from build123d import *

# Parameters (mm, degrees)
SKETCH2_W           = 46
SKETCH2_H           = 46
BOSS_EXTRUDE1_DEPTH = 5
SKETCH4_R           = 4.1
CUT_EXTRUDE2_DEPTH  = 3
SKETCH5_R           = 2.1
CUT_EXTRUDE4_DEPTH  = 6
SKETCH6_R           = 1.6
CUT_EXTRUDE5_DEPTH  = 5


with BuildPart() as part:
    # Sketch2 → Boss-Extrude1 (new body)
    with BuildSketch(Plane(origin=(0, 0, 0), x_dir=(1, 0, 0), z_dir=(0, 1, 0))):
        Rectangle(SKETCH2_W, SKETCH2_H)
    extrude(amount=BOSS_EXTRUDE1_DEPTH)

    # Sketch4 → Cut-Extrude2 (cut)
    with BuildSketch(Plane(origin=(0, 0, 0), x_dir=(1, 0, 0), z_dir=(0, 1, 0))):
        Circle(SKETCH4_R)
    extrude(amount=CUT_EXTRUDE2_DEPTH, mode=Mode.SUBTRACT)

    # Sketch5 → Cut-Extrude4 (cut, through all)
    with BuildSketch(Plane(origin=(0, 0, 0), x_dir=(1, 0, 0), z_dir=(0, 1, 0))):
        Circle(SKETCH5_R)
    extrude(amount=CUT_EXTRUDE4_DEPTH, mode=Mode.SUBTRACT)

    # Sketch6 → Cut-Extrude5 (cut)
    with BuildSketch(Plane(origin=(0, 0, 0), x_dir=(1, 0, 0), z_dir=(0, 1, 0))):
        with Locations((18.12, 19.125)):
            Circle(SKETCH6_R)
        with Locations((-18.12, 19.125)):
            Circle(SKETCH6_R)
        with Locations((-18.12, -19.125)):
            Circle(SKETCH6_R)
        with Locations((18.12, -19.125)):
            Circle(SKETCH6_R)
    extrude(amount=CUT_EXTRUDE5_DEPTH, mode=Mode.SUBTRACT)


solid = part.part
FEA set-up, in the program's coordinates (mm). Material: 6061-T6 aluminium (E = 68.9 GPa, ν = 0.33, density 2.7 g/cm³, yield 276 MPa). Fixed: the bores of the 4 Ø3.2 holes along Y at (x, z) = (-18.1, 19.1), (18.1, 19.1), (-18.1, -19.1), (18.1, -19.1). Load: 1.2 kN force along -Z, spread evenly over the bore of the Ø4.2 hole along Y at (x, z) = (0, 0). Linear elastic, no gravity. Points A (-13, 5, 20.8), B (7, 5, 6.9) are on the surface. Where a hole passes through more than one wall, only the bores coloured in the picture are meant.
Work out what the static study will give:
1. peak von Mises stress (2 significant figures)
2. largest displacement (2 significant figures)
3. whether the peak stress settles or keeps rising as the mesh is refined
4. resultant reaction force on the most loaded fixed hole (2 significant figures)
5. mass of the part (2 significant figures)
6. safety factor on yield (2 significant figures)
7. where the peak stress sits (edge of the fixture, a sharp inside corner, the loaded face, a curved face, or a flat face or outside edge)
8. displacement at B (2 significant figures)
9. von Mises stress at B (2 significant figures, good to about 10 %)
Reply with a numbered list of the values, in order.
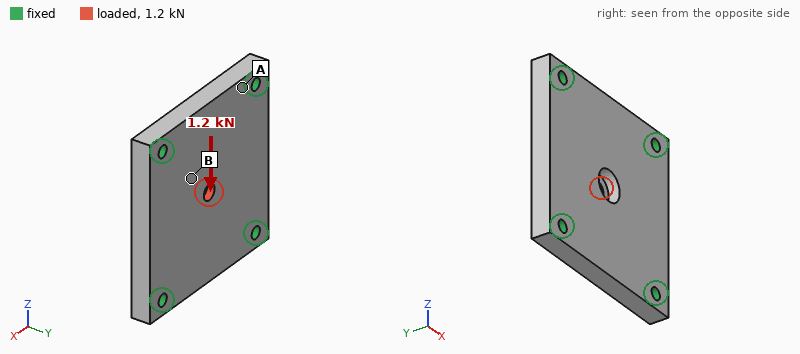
1. 82 MPa
2. 5.3 µm
3. settles
4. 340 N
5. 28 g
6. 3.4
7. the loaded face
8. 2.0 µm
9. 10 MPa
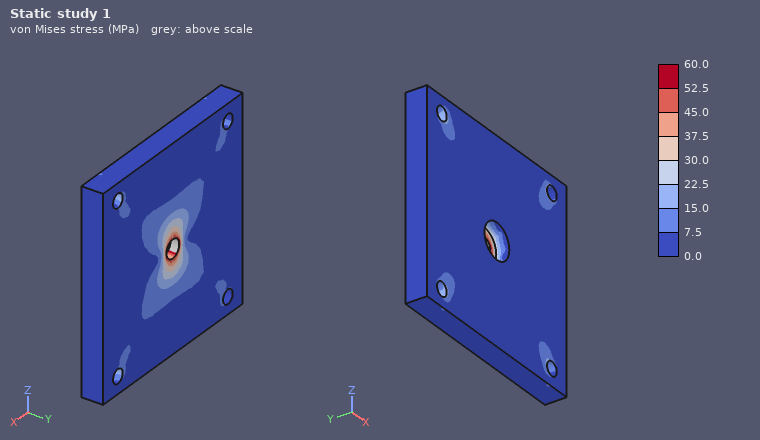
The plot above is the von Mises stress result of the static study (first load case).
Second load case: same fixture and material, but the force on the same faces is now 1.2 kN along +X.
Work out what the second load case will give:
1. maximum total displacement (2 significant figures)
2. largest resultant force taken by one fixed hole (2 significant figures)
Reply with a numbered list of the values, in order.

1. 5.4 µm
2. 340 N
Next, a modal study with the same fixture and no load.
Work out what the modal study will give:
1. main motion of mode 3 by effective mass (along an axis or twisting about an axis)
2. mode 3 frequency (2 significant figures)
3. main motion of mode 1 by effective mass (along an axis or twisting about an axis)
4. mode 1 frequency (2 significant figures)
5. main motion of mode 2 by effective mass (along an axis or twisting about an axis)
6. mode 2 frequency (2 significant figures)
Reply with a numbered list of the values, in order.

1. twisting about X
2. 19 kHz
3. along Y
4. 12 kHz
5. twisting about Z
6. 18 kHz
